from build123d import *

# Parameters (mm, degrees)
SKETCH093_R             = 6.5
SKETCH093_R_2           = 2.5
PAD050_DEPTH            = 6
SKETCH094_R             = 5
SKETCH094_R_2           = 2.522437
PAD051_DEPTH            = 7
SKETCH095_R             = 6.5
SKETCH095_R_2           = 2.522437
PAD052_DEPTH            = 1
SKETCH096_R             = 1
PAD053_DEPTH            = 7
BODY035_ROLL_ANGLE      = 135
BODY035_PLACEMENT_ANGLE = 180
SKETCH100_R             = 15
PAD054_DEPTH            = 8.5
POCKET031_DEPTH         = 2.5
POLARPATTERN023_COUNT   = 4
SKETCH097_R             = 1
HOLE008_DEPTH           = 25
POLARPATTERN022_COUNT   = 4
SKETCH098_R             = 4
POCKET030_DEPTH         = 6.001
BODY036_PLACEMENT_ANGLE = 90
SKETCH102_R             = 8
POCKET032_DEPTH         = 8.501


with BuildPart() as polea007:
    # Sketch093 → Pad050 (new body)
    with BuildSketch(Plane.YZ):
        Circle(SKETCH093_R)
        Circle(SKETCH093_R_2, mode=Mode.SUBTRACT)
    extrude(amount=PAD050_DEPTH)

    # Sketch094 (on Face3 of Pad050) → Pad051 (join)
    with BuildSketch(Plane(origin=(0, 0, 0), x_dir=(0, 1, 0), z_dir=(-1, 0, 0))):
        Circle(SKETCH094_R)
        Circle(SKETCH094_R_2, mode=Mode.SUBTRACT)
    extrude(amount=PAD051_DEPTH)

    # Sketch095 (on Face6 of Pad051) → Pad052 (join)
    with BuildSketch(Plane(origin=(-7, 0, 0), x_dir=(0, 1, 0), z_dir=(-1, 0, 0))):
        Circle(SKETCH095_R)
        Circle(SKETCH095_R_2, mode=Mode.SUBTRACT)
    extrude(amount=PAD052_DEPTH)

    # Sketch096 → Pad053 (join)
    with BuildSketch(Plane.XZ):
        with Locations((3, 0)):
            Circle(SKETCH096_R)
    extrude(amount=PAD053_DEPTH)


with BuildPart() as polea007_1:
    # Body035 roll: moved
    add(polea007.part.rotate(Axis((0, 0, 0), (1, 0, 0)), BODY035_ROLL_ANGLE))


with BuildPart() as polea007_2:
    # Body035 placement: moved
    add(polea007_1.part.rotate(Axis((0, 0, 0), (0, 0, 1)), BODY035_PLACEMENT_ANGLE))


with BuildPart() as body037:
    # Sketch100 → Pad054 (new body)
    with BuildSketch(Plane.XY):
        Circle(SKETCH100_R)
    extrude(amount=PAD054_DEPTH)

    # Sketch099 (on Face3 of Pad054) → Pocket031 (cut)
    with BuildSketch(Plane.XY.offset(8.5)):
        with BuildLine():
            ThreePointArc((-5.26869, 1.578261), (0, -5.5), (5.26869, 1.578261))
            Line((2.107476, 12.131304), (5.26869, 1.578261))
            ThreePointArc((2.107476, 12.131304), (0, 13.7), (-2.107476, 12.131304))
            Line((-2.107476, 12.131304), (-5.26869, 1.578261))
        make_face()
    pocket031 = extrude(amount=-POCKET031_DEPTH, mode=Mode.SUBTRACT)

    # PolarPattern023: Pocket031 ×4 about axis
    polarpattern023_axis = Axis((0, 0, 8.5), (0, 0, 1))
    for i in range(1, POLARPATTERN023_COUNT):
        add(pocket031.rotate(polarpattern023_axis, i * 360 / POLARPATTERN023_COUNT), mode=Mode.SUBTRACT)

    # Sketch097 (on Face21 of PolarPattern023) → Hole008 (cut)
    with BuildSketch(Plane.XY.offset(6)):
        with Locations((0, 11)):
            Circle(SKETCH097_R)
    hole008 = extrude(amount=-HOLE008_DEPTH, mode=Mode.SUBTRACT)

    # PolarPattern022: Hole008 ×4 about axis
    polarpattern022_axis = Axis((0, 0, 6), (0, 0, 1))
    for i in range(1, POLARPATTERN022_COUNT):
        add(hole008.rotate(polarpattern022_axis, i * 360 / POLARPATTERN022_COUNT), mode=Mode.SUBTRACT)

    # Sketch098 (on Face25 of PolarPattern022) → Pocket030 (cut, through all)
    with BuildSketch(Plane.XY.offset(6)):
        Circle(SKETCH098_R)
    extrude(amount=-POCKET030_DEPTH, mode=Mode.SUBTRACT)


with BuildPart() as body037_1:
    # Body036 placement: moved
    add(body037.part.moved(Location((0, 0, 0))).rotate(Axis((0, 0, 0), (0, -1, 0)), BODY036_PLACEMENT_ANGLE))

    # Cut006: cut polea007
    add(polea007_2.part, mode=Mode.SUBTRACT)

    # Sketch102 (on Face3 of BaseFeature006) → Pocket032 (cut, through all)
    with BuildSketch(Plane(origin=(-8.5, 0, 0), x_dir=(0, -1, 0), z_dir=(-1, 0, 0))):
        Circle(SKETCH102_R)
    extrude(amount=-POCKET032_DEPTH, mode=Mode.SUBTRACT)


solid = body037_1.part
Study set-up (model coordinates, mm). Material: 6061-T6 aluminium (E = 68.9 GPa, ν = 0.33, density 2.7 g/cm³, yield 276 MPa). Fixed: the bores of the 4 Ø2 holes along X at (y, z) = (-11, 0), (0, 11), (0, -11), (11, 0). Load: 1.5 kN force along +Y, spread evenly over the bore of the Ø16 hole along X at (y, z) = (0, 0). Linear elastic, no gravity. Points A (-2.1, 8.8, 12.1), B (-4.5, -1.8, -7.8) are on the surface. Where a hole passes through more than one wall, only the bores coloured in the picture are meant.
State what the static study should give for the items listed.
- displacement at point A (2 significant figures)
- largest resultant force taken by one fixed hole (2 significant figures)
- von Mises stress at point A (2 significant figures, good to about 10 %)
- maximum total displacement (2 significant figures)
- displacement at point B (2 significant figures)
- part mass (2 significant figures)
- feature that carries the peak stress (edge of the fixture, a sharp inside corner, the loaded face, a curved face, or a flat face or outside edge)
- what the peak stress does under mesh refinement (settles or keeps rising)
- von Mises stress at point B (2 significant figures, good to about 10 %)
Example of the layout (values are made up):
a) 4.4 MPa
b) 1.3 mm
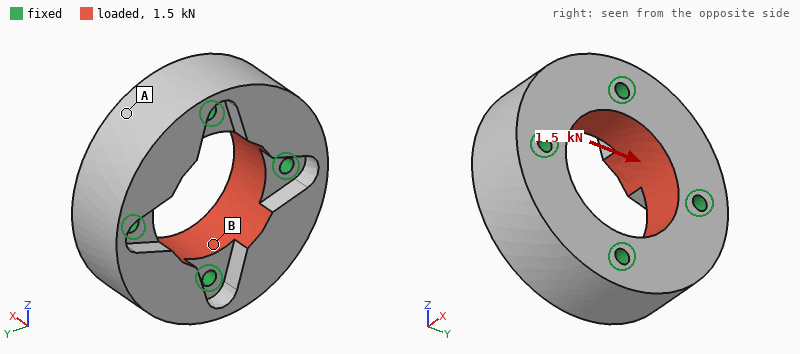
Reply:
a) 0.55 µm
b) 420 N
c) 3.5 MPa
d) 1.2 µm
e) 0.78 µm
f) 11 g
g) edge of the fixture
h) keeps rising
i) 8.0 MPa
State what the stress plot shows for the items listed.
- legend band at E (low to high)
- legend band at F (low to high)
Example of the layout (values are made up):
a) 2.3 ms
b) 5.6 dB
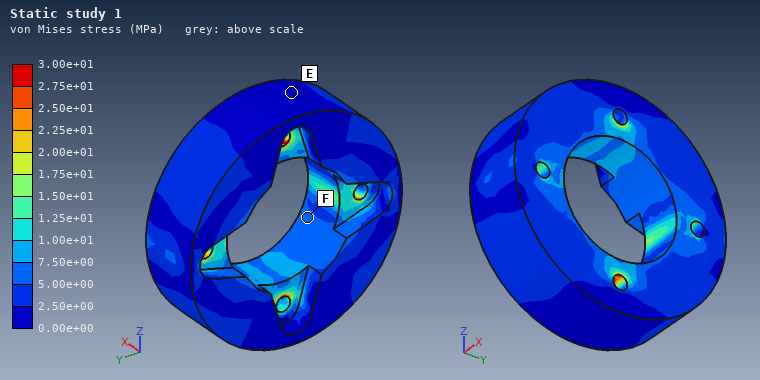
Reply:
a) 0.00e+00 to 2.50e+00 MPa
b) 5.00e+00 to 7.50e+00 MPa
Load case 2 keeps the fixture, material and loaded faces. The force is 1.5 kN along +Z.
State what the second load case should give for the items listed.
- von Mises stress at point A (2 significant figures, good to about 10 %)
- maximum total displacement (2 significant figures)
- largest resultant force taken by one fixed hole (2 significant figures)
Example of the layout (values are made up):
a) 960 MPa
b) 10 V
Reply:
a) 4.0 MPa
b) 1.2 µm
c) 420 N
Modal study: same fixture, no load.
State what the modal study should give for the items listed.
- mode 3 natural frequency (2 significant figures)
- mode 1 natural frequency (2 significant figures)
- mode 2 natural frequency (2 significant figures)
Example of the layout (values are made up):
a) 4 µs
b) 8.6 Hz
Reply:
a) 45 kHz
b) 41 kHz
c) 45 kHz
